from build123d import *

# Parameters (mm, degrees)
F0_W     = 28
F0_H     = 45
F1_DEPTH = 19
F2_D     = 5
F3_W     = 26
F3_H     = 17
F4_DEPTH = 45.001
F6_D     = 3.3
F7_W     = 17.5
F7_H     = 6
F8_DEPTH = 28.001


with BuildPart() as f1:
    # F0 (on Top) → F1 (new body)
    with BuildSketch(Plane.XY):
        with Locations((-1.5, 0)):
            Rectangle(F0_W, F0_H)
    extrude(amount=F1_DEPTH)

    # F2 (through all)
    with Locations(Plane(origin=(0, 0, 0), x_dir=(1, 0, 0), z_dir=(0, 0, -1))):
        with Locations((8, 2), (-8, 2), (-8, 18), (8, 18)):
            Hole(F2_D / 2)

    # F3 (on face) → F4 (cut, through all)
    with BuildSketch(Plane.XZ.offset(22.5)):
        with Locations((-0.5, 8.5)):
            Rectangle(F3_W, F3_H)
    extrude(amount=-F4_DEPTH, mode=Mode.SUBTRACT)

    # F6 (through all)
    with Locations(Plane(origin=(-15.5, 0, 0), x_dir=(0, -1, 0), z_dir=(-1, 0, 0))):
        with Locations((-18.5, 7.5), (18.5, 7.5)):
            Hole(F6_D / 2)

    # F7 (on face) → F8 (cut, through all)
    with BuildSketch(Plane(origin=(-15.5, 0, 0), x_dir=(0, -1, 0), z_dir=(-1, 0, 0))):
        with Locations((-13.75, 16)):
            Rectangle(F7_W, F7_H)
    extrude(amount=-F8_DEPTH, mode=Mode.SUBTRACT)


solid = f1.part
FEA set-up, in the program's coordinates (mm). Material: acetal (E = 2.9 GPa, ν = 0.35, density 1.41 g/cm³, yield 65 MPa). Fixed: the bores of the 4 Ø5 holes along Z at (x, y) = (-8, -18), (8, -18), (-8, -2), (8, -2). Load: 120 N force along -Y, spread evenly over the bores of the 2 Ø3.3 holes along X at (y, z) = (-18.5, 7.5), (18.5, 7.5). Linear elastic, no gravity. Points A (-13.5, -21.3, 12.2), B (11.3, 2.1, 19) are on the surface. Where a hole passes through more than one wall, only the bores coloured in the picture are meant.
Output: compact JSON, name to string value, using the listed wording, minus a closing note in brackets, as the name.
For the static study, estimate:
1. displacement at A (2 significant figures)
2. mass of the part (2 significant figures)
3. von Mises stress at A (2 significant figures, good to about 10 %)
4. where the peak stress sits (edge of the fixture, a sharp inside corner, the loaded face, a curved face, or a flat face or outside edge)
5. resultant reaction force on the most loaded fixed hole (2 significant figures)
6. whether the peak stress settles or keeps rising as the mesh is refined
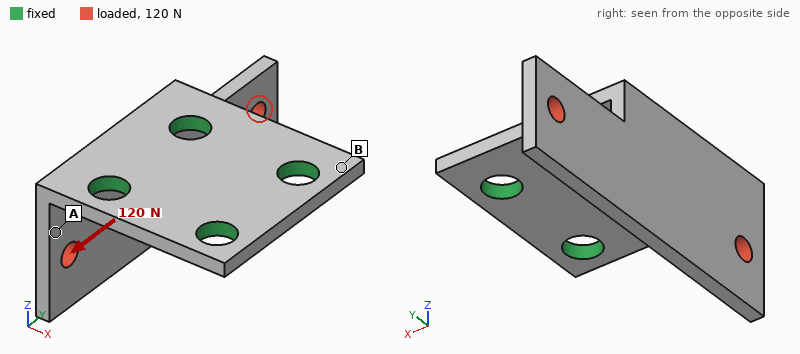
{"displacement at A": "0.18 mm", "mass of the part": "3.9 g", "von Mises stress at A": "8.1 MPa", "where the peak stress sits": "edge of the fixture", "resultant reaction force on the most loaded fixed hole": "100 N", "whether the peak stress settles or keeps rising as the mesh is refined": "keeps rising"}
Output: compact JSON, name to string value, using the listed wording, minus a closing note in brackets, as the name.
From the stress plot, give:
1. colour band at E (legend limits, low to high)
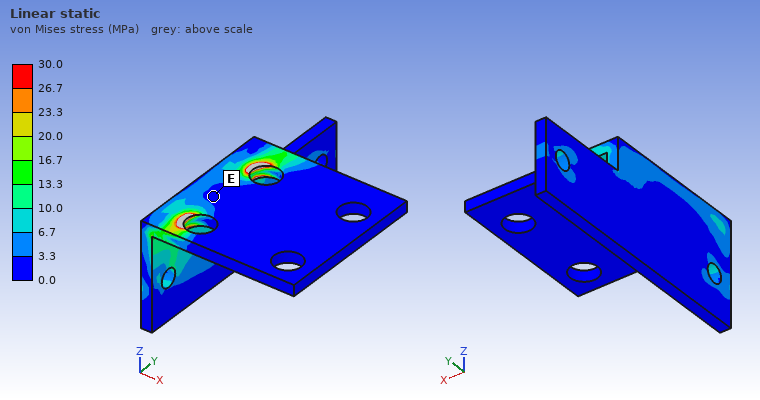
{"colour band at E": "0.0 to 3.3 MPa"}
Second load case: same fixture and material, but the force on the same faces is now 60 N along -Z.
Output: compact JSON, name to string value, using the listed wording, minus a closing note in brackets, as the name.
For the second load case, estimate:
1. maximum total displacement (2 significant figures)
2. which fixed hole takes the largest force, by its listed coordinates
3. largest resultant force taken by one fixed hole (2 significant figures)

{"maximum total displacement": "0.59 mm", "which fixed hole takes the largest force, by its listed coordinates": "(-8, -2)", "largest resultant force taken by one fixed hole": "64 N"}
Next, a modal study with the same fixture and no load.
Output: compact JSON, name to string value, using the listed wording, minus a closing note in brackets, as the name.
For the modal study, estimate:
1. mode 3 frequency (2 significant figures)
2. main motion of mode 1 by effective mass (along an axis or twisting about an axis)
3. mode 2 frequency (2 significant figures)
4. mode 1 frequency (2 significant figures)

{"mode 3 frequency": "1900 Hz", "main motion of mode 1 by effective mass": "along X", "mode 2 frequency": "1100 Hz", "mode 1 frequency": "600 Hz"}
